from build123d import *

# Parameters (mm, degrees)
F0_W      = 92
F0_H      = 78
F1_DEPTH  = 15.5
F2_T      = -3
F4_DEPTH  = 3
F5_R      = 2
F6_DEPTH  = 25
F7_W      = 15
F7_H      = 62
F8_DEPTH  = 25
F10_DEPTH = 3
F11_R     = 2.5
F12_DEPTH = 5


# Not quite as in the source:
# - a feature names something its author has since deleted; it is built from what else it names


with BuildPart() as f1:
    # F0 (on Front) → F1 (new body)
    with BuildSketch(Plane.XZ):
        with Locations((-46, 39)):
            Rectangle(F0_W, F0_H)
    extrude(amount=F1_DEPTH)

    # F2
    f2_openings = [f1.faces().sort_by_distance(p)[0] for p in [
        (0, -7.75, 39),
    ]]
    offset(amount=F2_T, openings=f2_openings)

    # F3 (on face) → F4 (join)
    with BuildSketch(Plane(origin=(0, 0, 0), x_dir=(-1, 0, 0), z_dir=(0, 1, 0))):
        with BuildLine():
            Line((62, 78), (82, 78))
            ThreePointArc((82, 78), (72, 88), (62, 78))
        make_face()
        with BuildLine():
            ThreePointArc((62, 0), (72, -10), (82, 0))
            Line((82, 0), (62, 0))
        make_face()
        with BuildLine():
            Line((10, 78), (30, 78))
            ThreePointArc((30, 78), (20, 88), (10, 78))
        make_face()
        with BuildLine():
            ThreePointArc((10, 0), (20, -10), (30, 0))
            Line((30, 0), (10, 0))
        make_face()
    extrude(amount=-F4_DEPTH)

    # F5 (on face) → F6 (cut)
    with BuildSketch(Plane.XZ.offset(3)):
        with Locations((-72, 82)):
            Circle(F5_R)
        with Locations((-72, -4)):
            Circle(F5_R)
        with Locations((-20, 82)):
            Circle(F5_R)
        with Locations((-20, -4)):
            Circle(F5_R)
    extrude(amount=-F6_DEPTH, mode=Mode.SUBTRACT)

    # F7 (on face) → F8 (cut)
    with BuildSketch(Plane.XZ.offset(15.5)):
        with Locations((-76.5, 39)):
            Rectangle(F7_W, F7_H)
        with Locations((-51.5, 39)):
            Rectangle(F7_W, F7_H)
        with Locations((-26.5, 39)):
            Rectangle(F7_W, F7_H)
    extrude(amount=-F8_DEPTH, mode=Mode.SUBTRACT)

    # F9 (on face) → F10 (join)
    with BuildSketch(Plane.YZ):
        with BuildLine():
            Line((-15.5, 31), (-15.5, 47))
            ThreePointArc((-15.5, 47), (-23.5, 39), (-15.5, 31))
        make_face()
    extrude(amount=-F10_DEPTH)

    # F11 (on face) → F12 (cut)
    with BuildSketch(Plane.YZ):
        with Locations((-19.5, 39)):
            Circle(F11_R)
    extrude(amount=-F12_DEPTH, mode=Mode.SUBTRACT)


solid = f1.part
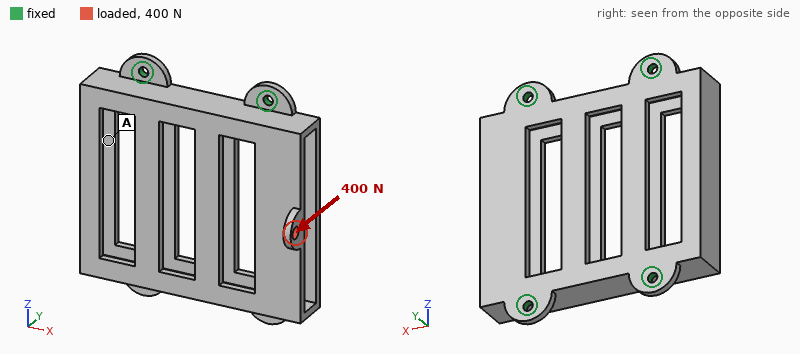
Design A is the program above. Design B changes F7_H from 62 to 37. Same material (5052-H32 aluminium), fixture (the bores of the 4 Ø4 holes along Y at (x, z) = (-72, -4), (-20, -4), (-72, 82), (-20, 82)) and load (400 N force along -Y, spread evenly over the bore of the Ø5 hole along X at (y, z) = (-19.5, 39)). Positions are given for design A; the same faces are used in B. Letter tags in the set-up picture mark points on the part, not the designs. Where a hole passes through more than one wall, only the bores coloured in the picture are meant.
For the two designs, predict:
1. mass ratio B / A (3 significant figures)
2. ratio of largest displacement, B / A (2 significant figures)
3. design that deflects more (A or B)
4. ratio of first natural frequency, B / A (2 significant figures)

1.19
0.91
A
1.1
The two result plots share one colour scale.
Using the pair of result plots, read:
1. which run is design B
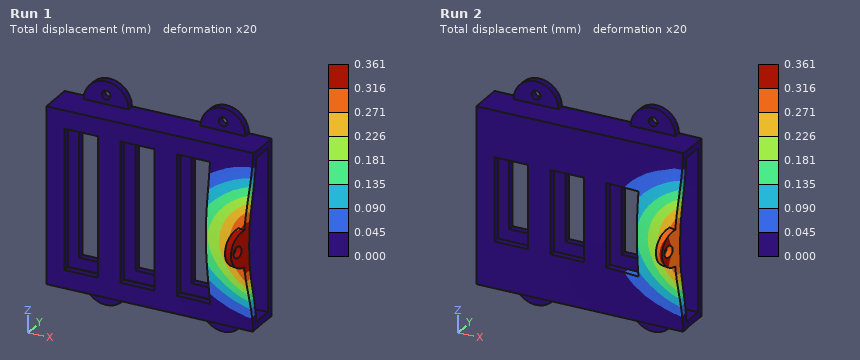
Run 2
